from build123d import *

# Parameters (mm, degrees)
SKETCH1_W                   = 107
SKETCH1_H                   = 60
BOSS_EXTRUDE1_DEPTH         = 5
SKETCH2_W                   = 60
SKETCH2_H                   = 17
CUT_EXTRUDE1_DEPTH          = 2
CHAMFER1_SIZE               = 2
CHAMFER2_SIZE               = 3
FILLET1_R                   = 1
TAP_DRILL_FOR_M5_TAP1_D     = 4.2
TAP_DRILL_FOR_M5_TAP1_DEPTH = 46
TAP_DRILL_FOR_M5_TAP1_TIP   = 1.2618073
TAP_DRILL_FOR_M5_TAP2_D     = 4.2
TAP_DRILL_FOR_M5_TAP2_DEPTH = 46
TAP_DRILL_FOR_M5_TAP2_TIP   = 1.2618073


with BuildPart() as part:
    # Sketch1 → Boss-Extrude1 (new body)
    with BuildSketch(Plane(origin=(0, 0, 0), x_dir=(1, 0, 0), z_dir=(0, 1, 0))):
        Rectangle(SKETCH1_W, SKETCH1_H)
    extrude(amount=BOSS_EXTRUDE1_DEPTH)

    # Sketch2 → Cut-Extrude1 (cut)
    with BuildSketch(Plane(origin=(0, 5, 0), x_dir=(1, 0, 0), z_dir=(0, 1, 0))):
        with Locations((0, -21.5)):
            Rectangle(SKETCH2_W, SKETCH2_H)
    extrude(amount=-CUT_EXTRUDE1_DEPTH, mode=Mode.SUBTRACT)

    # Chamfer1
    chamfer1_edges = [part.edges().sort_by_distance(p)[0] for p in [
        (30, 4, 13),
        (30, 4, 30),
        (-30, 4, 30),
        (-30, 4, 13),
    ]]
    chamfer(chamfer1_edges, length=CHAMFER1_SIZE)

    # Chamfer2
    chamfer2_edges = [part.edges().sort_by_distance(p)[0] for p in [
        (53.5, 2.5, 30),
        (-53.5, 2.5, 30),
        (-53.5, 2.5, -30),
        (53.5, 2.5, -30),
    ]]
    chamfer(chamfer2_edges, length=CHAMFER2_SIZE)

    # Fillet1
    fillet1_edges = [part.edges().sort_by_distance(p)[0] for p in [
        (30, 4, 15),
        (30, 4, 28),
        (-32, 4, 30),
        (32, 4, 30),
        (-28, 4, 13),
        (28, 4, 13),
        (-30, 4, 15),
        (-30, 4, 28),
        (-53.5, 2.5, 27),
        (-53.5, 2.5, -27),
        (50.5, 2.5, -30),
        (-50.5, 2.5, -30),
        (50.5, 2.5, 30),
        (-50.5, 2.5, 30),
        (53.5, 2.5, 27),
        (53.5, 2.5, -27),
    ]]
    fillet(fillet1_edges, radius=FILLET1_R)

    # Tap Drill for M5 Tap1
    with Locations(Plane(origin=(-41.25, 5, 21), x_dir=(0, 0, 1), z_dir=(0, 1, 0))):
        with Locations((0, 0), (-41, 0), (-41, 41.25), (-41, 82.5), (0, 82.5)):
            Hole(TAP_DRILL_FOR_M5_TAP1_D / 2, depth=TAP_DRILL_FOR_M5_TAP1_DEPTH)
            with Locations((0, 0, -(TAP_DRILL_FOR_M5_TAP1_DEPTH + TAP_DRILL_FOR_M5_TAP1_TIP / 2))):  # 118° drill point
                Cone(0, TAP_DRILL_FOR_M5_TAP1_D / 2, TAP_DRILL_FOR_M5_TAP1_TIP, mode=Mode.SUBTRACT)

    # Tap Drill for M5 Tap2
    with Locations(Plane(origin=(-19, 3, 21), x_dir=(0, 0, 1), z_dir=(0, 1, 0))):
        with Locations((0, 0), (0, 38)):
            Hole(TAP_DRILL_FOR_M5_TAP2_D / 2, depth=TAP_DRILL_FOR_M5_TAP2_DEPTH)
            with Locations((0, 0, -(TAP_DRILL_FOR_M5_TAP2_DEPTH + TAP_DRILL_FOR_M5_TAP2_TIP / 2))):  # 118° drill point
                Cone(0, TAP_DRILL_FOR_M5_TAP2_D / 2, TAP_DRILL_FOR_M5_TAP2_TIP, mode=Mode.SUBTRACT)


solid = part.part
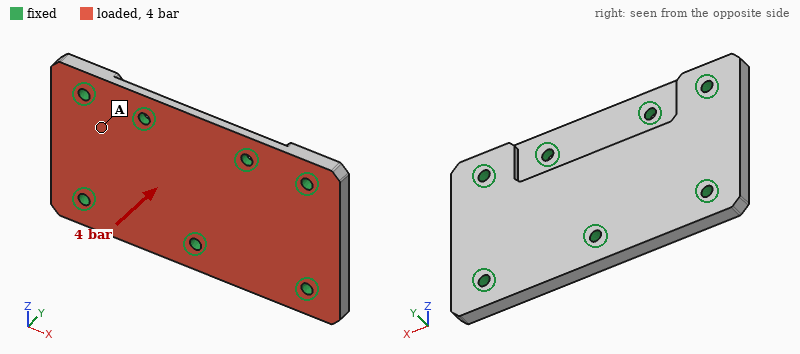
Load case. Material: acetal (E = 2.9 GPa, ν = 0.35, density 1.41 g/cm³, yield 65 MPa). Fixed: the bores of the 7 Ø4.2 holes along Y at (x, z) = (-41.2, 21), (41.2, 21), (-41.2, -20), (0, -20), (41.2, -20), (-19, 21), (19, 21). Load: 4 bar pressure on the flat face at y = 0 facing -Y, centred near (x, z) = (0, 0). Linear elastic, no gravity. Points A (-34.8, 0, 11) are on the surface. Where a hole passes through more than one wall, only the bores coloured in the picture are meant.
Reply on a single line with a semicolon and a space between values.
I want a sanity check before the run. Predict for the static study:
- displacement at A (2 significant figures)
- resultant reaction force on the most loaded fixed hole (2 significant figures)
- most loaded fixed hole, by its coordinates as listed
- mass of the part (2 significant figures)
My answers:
0.098 mm; 540 N; (0, -20); 42 g
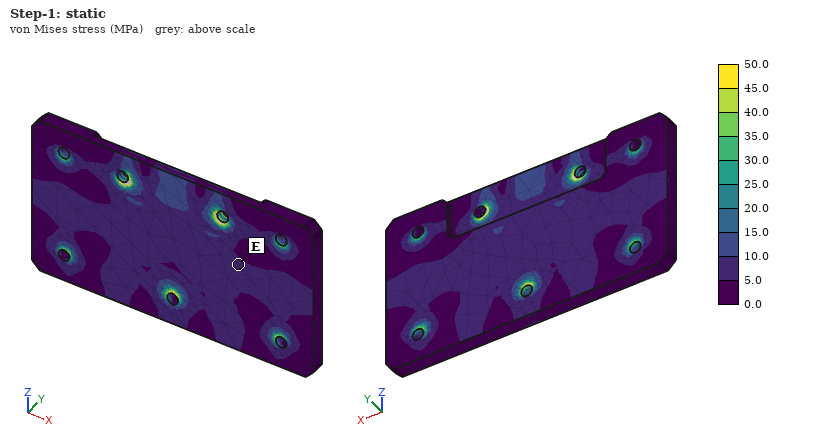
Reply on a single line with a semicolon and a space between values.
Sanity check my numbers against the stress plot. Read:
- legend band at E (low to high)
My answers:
5.0 to 10.0 MPa
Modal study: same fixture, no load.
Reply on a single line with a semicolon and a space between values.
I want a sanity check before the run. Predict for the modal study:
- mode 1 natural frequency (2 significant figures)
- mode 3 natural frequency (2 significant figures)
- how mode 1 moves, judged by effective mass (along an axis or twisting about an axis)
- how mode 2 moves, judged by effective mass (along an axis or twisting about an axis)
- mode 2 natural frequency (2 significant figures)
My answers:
2800 Hz; 3500 Hz; along Y; twisting about Z; 3300 Hz
